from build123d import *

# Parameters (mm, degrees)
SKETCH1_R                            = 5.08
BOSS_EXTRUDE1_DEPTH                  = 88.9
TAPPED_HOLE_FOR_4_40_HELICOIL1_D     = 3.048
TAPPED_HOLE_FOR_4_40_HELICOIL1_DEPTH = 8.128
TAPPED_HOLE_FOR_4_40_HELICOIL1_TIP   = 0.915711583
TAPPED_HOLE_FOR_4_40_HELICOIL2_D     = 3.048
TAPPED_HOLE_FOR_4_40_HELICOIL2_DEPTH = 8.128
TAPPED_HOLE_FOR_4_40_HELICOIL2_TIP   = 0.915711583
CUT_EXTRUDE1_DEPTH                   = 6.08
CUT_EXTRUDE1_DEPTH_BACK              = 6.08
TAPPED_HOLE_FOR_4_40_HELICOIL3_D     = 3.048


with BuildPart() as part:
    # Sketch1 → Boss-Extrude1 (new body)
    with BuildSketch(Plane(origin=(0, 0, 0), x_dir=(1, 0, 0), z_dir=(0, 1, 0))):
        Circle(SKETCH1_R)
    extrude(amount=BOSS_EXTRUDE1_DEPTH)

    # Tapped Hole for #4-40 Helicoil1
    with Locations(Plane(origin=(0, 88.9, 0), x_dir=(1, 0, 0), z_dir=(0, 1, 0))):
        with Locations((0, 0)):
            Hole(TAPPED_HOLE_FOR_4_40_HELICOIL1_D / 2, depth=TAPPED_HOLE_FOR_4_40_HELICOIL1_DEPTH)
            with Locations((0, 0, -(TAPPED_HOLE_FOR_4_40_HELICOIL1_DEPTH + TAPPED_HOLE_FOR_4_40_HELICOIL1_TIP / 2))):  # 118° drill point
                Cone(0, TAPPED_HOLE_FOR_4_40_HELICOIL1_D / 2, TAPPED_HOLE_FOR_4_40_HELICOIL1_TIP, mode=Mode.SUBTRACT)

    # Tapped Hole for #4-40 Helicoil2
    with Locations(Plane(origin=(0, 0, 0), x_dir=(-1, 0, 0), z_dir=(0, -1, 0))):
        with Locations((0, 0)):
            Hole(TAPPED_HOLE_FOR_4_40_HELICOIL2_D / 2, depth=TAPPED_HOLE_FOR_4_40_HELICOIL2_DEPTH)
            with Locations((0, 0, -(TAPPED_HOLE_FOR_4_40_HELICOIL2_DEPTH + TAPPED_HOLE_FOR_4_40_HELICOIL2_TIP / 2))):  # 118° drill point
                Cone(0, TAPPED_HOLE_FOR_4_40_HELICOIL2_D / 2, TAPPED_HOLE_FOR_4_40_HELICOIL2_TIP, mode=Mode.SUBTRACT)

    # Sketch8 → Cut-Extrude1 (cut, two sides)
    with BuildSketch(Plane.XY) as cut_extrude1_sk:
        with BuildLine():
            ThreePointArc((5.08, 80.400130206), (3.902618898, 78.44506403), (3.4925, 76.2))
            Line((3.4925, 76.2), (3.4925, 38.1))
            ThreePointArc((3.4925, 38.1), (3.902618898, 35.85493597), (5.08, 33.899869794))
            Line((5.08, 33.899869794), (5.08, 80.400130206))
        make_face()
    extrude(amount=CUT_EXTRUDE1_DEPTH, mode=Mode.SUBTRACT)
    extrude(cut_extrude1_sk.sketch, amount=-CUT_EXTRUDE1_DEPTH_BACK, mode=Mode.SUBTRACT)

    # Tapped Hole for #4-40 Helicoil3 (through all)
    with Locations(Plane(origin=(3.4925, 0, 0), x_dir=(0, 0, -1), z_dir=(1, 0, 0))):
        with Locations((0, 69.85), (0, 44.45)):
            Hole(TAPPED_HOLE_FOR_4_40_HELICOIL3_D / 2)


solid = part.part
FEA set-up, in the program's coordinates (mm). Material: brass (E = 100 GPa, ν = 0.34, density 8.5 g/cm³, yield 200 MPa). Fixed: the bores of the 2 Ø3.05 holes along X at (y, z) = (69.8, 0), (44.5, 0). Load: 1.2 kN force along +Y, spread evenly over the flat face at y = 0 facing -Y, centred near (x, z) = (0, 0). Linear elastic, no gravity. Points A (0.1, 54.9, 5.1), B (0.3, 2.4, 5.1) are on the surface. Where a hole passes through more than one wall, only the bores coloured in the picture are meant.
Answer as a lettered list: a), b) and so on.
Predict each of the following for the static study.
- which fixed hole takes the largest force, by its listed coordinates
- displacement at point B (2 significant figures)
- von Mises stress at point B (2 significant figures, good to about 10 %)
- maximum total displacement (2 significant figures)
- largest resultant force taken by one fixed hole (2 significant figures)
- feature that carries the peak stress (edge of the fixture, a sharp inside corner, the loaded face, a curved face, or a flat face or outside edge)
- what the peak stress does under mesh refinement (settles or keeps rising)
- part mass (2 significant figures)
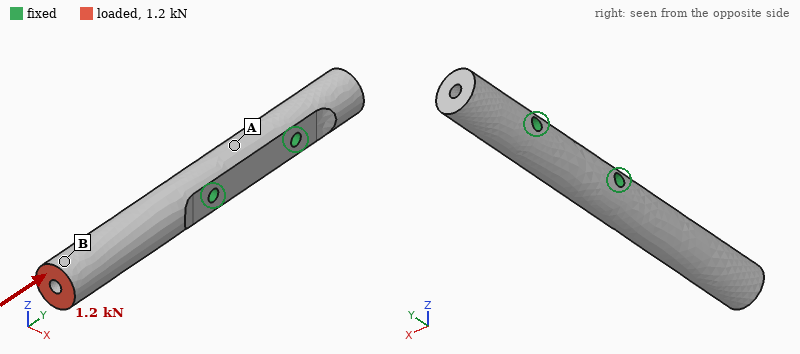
a) (44.5, 0)
b) 8.8 µm
c) 16 MPa
d) 10 µm
e) 1.2 kN
f) edge of the fixture
g) keeps rising
h) 56 g
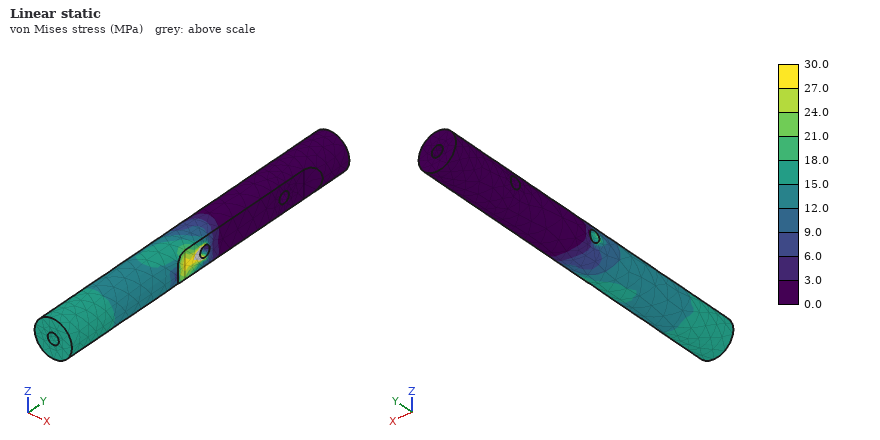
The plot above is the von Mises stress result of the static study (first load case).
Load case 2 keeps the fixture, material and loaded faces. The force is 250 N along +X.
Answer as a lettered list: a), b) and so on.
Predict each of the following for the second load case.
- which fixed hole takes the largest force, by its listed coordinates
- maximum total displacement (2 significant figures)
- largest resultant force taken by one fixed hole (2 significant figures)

a) (44.5, 0)
b) 0.17 mm
c) 280 N
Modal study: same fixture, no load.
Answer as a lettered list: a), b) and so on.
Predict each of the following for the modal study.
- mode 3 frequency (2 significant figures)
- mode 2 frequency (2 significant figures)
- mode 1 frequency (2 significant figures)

a) 10000 Hz
b) 2300 Hz
c) 2200 Hz
